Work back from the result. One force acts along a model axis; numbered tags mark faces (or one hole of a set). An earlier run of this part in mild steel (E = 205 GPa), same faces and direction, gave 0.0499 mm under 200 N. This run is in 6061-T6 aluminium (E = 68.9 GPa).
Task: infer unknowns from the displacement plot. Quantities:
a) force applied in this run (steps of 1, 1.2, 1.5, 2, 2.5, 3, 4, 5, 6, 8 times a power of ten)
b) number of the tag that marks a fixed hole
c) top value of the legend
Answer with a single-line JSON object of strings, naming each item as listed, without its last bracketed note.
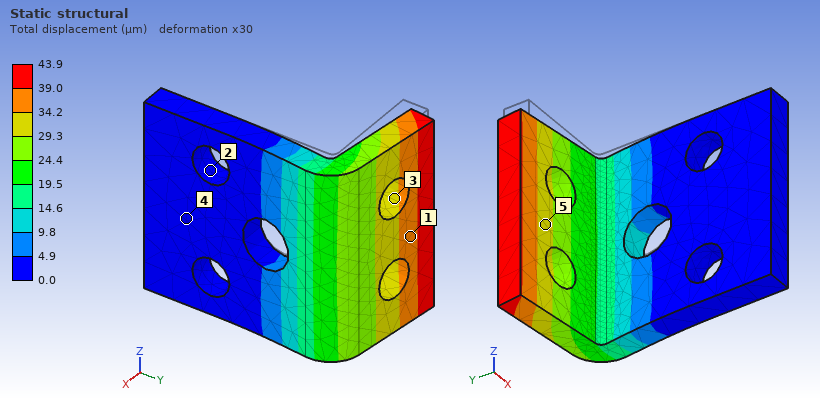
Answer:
{"force applied in this run": "60 N", "number of the tag that marks a fixed hole": "2", "top value of the legend": "43.9 µm"}
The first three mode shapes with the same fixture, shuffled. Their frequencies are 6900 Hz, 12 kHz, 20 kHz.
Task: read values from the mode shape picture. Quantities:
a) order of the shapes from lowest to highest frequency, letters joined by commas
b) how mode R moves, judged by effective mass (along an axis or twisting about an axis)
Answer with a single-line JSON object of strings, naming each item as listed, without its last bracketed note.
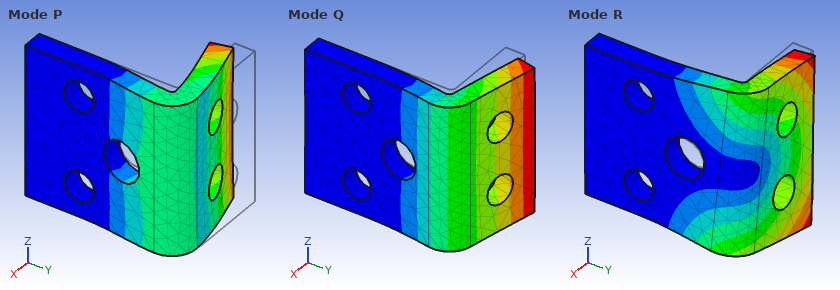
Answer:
{"order of the shapes from lowest to highest frequency, letters joined by commas": "Q, R, P", "how mode R moves, judged by effective mass": "along Z"}
